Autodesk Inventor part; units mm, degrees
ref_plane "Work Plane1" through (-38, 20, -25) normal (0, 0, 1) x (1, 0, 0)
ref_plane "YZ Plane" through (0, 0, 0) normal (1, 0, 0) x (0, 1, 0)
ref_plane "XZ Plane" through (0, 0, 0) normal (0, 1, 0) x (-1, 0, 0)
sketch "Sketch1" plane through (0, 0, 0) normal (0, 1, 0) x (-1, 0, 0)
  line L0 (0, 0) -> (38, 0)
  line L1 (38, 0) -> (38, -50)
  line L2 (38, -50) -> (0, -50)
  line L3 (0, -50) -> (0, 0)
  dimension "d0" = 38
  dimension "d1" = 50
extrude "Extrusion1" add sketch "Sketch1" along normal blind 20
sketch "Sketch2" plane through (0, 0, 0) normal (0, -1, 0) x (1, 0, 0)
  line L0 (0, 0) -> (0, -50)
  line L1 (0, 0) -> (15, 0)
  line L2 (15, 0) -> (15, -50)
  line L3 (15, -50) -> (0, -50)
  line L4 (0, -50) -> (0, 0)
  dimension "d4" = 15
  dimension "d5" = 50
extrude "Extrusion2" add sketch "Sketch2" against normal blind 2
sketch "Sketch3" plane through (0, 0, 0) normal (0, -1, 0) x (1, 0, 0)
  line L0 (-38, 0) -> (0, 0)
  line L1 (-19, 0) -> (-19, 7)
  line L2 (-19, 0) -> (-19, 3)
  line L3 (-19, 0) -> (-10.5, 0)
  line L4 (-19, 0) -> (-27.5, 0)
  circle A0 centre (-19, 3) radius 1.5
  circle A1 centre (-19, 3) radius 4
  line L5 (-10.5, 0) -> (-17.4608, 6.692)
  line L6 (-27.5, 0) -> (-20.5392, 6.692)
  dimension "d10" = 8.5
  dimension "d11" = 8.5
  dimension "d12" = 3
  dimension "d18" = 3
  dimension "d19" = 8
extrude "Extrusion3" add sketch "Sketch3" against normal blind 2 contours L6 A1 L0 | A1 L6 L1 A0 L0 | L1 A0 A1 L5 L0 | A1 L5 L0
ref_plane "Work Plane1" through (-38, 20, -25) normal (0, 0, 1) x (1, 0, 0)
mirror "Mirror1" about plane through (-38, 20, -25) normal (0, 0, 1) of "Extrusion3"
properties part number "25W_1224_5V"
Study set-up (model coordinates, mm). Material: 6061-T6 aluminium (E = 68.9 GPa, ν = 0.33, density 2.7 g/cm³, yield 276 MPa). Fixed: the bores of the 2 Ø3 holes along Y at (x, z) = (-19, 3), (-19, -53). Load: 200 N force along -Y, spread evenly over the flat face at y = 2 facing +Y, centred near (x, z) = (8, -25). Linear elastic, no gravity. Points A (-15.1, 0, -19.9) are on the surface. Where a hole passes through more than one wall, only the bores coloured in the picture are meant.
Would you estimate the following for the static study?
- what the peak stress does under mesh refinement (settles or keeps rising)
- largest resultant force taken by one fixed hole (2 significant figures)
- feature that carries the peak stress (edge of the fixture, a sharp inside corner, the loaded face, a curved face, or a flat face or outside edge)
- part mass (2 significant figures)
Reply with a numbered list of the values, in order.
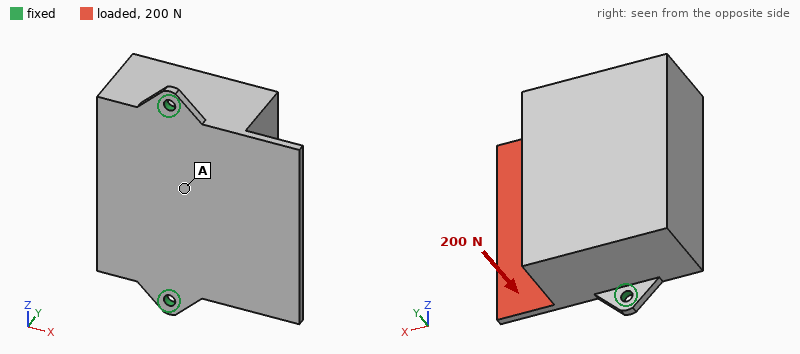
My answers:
1. keeps rising
2. 120 N
3. edge of the fixture
4. 110 g
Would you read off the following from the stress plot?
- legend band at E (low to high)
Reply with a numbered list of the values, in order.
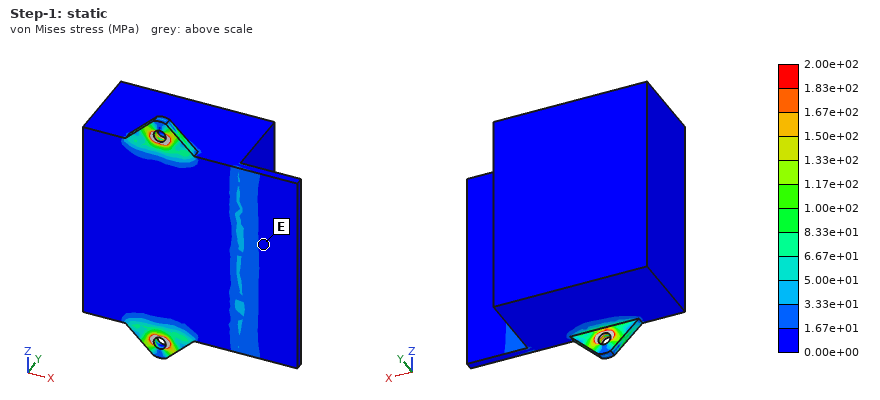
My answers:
1. 0.00e+00 to 1.67e+01 MPa
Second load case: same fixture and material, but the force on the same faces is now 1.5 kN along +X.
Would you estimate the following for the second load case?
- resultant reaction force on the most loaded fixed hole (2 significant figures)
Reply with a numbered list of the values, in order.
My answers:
1. 750 N
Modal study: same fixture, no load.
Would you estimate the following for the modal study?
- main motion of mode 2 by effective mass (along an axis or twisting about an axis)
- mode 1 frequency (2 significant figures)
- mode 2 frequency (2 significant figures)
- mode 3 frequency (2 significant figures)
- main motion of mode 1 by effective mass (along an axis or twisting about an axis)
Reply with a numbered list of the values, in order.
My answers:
1. along Y
2. 840 Hz
3. 5000 Hz
4. 6900 Hz
5. along X
